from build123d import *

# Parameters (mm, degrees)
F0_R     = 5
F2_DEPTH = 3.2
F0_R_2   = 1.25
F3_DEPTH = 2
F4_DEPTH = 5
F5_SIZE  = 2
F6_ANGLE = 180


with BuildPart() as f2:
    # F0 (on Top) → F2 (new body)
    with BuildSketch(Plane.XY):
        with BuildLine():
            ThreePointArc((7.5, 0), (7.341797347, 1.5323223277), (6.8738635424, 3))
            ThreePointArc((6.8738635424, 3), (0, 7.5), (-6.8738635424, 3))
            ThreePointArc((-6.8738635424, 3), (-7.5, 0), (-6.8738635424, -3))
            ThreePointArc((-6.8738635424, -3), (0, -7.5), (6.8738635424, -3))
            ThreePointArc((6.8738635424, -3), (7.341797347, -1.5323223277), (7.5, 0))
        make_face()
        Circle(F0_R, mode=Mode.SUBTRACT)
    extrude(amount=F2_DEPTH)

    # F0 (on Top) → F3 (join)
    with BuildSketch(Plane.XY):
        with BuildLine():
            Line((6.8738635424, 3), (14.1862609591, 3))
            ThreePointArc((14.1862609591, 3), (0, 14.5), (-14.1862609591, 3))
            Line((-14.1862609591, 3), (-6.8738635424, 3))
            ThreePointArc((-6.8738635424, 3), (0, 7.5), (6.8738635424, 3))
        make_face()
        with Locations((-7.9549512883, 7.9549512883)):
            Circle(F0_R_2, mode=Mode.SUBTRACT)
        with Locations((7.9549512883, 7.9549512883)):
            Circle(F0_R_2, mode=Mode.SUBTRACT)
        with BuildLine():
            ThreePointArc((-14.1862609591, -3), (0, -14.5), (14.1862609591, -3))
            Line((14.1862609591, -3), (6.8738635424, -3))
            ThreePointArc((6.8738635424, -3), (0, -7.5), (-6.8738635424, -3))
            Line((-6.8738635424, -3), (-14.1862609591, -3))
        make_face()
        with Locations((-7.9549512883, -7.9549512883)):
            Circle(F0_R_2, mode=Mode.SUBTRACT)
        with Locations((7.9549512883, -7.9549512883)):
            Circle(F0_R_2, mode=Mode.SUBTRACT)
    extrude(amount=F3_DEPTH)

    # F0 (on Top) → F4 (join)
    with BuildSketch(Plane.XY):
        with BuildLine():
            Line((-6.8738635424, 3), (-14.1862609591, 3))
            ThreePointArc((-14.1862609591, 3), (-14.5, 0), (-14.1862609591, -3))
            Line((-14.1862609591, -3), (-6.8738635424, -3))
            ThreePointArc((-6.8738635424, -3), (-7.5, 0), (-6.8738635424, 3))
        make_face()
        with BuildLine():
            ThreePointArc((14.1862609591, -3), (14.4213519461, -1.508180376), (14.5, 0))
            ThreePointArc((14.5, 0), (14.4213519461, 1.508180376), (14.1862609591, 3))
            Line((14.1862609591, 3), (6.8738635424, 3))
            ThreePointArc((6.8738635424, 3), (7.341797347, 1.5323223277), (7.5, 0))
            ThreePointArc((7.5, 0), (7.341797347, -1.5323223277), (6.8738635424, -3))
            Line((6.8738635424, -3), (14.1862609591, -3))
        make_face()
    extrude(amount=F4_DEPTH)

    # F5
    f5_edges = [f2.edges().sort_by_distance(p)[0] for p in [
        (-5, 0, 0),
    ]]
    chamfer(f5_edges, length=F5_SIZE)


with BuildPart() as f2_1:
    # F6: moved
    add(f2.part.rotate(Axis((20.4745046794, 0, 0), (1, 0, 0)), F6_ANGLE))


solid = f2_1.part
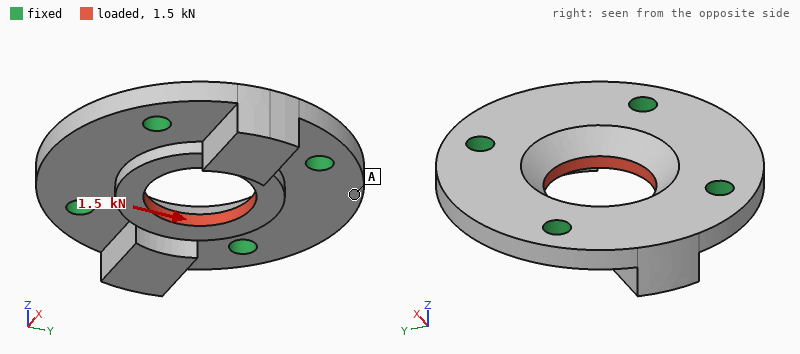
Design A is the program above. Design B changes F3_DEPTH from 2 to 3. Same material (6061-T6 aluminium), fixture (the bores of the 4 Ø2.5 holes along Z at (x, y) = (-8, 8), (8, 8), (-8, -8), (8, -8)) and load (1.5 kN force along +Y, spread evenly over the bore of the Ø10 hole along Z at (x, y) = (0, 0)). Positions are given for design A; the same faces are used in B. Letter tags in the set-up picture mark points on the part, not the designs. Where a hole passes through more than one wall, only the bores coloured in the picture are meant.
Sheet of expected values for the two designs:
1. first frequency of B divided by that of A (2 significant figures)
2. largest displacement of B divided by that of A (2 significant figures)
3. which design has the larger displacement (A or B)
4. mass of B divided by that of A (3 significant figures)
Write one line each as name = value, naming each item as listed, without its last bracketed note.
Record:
first frequency of B divided by that of A = 1.4
largest displacement of B divided by that of A = 0.55
which design has the larger displacement = A
mass of B divided by that of A = 1.27
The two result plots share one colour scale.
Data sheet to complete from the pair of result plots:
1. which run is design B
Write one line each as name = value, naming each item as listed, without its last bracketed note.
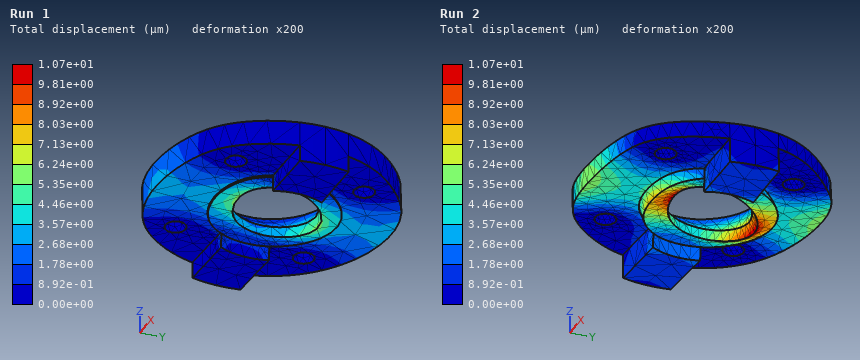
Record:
which run is design B = Run 1
